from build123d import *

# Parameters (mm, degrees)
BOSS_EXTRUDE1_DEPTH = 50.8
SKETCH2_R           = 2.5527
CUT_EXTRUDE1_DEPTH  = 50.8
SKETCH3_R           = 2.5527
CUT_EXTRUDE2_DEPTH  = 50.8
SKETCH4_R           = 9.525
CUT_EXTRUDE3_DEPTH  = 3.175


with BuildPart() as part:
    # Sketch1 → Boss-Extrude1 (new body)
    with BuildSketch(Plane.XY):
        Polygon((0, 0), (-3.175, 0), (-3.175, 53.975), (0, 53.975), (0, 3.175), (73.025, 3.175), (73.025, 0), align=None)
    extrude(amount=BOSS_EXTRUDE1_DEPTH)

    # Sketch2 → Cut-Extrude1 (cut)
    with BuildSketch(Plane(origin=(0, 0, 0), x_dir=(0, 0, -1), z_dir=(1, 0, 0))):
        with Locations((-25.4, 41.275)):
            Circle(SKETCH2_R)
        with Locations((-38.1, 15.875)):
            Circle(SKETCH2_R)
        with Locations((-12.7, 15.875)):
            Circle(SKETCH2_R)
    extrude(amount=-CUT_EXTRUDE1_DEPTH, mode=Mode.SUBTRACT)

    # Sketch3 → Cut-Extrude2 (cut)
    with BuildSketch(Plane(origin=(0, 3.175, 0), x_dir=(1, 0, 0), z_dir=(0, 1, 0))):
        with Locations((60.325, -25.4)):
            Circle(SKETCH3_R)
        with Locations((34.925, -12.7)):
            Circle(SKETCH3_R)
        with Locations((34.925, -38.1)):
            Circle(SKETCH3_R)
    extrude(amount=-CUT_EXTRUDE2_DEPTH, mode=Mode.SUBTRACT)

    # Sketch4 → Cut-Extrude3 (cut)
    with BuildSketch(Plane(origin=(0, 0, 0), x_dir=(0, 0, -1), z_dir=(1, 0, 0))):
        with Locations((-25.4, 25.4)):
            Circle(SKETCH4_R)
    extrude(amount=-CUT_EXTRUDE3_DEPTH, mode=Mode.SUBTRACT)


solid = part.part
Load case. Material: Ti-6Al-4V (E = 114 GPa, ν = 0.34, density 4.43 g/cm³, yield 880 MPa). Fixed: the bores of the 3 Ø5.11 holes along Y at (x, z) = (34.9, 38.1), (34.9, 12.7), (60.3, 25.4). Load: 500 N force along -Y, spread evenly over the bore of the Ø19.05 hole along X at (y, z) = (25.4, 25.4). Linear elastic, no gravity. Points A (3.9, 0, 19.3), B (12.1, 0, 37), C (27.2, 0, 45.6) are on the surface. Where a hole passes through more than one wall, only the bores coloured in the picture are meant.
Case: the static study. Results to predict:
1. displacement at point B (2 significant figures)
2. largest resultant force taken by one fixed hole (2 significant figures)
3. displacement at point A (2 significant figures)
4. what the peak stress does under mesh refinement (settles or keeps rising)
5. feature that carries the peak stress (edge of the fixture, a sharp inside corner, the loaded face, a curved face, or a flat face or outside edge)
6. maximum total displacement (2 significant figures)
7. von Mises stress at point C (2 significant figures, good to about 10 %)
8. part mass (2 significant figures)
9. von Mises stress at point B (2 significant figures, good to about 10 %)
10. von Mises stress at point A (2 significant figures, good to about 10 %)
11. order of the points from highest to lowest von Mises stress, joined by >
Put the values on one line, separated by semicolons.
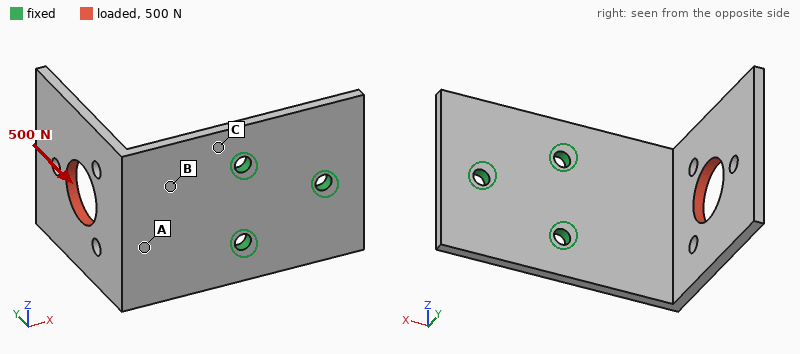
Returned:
0.22 mm; 290 N; 0.37 mm; keeps rising; edge of the fixture; 1.1 mm; 150 MPa; 85 g; 71 MPa; 31 MPa; C > B > A
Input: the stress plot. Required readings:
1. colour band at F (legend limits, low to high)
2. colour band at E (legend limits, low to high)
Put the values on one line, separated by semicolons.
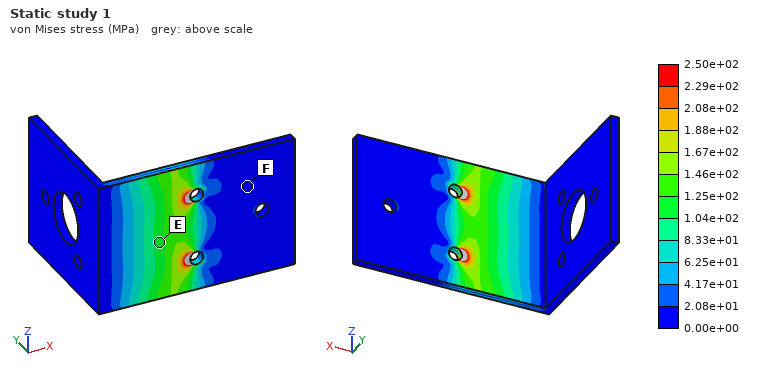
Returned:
0.00e+00 to 2.08e+01 MPa; 1.04e+02 to 1.25e+02 MPa
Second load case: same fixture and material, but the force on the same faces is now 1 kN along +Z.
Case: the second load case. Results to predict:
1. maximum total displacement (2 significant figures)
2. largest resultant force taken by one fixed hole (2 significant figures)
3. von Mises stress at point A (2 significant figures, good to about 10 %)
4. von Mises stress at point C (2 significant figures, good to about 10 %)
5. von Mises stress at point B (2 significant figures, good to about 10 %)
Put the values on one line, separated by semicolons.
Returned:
1.3 mm; 1.4 kN; 140 MPa; 170 MPa; 150 MPa
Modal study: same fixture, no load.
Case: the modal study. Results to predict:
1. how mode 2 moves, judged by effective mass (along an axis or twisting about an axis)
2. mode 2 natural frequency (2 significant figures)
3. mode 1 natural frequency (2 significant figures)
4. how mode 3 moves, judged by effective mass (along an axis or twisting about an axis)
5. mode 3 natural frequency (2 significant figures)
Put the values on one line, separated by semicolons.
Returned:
along Z; 830 Hz; 460 Hz; along Y; 1300 Hz
